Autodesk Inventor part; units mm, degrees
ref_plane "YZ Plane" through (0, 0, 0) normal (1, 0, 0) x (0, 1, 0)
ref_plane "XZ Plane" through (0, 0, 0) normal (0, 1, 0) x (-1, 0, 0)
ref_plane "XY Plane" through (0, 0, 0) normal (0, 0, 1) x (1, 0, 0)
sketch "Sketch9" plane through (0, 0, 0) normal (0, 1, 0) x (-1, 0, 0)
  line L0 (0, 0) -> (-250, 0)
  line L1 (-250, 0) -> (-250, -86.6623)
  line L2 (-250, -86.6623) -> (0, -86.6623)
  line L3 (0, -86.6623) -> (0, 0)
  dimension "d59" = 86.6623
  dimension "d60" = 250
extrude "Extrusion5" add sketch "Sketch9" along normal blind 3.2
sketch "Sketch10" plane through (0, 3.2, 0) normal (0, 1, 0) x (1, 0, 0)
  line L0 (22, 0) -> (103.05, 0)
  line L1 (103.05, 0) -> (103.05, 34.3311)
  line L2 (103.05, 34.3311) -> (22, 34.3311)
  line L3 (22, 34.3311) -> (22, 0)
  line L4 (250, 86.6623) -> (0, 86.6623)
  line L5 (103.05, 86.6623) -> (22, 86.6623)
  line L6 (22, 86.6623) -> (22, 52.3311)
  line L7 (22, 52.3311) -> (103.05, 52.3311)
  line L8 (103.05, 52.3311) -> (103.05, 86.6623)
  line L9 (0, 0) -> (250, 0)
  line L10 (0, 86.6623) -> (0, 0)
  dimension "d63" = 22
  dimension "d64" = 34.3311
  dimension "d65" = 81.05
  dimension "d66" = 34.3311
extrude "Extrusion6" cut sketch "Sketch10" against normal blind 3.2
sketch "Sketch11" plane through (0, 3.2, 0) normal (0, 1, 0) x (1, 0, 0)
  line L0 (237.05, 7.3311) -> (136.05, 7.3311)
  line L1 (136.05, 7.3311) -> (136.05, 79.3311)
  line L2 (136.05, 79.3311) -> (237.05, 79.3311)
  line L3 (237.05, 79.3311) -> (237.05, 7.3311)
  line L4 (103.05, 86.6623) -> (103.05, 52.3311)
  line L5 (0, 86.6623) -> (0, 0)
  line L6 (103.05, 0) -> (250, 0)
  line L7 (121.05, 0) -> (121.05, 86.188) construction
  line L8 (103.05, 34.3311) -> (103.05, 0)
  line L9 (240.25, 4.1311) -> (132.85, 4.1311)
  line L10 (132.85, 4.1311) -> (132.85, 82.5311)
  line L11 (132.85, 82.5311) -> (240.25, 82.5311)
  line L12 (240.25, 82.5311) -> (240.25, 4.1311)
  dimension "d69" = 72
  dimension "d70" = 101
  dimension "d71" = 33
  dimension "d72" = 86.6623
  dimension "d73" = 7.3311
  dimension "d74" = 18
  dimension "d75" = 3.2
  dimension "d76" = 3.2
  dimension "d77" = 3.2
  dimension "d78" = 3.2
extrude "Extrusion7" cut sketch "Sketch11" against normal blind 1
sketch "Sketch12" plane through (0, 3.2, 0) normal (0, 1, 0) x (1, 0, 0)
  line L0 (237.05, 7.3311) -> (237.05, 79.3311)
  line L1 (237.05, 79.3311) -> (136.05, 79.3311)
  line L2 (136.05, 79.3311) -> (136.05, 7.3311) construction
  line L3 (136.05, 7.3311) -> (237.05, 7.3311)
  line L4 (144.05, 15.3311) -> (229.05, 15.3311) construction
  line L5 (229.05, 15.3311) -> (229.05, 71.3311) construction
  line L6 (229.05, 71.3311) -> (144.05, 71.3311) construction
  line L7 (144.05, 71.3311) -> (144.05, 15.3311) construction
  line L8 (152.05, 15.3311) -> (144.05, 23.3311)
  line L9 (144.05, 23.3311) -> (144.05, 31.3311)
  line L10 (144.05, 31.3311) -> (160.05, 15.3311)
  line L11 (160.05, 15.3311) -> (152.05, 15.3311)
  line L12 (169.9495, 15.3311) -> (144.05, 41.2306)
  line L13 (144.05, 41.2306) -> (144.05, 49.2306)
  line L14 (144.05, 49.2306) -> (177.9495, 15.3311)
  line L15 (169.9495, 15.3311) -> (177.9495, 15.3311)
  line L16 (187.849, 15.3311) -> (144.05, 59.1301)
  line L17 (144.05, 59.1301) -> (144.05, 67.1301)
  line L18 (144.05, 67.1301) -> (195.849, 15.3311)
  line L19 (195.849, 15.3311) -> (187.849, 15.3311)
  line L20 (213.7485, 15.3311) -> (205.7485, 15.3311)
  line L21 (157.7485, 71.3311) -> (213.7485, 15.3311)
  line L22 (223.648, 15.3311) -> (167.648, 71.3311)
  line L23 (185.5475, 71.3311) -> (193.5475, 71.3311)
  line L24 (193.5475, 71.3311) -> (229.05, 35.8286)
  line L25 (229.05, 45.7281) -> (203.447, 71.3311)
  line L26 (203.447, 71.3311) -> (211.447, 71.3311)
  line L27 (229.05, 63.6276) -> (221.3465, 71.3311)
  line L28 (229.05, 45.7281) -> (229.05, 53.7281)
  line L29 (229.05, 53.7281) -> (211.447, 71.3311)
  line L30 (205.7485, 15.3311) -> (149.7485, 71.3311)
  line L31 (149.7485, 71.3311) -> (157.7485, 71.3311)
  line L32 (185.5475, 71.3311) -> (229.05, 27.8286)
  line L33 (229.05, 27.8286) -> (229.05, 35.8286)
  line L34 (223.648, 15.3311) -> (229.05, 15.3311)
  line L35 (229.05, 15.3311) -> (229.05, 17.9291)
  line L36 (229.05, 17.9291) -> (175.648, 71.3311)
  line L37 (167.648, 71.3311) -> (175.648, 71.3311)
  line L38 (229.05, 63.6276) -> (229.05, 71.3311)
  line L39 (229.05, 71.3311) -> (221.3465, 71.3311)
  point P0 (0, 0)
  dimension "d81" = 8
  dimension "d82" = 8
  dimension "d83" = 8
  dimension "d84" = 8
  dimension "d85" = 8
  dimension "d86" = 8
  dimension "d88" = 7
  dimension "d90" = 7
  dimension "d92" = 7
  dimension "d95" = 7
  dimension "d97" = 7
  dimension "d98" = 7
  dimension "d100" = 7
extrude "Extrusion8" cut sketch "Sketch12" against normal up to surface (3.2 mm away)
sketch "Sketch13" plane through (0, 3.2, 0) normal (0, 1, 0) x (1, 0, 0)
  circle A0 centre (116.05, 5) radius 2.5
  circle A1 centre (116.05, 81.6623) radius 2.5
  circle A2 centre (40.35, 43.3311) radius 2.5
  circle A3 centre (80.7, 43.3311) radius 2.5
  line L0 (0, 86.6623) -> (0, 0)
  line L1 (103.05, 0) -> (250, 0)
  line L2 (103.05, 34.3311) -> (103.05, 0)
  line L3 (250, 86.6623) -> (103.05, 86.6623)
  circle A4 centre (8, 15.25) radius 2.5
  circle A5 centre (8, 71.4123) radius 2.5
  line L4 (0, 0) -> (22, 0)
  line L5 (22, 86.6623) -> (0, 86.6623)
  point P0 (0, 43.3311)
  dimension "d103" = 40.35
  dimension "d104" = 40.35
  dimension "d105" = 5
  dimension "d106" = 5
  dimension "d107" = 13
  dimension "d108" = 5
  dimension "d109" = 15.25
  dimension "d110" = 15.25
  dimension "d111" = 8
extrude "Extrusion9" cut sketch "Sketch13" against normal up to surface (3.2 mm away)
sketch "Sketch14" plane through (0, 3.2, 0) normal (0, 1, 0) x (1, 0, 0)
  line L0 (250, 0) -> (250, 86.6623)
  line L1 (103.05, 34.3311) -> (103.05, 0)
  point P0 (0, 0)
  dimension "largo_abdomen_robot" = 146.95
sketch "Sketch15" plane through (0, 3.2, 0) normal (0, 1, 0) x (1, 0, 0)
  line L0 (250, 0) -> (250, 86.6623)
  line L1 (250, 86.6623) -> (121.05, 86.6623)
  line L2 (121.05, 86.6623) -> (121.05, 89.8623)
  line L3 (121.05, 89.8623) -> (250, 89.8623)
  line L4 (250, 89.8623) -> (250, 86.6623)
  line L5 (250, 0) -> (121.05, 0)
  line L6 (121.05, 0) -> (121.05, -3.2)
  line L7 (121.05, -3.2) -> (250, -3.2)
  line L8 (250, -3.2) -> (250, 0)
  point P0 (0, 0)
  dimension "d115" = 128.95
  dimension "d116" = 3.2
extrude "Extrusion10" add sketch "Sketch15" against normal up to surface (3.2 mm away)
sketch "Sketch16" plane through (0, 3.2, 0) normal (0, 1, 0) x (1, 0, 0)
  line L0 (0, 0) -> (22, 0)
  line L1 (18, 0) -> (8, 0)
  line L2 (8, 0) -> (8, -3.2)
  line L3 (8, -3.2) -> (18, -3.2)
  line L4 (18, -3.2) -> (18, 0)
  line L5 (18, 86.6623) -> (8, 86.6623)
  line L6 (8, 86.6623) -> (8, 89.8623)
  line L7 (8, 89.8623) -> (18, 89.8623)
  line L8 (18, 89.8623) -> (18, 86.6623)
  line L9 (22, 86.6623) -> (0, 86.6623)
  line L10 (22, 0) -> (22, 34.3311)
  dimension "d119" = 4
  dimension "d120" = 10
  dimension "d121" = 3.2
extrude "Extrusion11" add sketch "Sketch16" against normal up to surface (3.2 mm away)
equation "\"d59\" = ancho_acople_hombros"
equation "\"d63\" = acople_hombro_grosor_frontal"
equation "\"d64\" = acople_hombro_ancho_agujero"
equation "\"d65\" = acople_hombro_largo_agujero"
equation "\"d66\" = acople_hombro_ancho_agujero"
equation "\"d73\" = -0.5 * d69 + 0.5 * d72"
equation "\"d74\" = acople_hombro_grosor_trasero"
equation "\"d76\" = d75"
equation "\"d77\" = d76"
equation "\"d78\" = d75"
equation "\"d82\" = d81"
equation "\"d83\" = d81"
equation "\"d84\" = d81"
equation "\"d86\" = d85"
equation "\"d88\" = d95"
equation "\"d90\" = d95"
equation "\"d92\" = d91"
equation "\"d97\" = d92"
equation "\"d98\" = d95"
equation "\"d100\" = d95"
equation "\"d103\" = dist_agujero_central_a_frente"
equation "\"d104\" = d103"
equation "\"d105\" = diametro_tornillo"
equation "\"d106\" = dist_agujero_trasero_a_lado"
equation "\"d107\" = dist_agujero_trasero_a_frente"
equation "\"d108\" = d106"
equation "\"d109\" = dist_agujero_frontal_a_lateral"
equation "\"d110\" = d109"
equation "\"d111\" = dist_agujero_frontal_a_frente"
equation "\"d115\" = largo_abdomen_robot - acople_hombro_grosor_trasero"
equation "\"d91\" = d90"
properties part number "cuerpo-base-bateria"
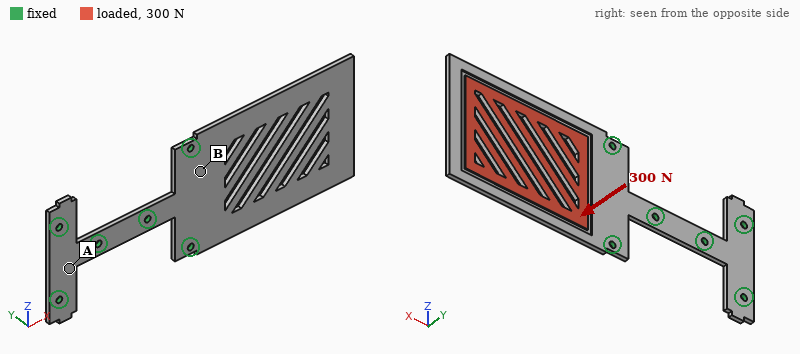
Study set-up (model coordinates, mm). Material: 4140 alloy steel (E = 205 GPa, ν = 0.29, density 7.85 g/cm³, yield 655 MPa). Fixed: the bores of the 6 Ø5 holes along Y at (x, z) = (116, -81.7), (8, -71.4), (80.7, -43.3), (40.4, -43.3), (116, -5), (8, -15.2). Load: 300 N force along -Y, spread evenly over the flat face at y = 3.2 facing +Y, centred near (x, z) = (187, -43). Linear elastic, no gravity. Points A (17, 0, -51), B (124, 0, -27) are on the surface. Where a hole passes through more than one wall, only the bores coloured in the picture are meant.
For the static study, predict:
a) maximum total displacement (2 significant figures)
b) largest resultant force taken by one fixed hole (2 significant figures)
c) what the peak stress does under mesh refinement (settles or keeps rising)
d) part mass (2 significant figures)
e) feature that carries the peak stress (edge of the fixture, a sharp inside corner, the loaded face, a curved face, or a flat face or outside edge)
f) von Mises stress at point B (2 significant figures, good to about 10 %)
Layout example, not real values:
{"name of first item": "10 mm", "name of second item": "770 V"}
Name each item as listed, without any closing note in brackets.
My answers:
{"maximum total displacement": "3.0 mm", "largest resultant force taken by one fixed hole": "230 N", "what the peak stress does under mesh refinement": "keeps rising", "part mass": "360 g", "feature that carries the peak stress": "edge of the fixture", "von Mises stress at point B": "83 MPa"}
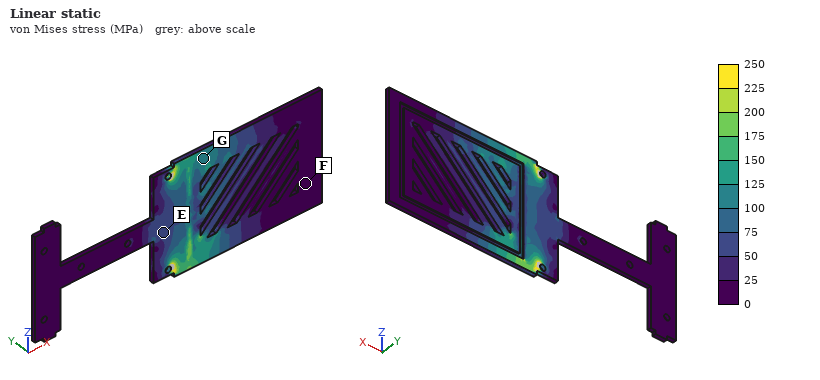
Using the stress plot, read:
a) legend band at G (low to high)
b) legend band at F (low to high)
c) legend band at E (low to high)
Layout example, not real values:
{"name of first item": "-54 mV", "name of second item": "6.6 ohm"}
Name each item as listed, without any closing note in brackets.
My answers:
{"legend band at G": "100 to 125 MPa", "legend band at F": "0 to 25 MPa", "legend band at E": "50 to 75 MPa"}
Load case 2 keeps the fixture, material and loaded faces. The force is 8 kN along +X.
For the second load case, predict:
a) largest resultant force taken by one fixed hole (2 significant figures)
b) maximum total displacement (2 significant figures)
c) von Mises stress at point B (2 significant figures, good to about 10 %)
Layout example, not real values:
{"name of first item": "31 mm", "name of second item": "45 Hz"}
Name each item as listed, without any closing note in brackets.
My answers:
{"largest resultant force taken by one fixed hole": "3.4 kN", "maximum total displacement": "2.9 mm", "von Mises stress at point B": "54 MPa"}
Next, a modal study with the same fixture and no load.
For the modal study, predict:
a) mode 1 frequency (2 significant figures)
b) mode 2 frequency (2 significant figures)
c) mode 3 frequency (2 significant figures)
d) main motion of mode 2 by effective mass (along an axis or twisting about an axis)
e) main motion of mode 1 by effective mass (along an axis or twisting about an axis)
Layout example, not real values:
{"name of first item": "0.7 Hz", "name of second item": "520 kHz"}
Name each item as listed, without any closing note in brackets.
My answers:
{"mode 1 frequency": "130 Hz", "mode 2 frequency": "380 Hz", "mode 3 frequency": "770 Hz", "main motion of mode 2 by effective mass": "twisting about X", "main motion of mode 1 by effective mass": "along Y"}
